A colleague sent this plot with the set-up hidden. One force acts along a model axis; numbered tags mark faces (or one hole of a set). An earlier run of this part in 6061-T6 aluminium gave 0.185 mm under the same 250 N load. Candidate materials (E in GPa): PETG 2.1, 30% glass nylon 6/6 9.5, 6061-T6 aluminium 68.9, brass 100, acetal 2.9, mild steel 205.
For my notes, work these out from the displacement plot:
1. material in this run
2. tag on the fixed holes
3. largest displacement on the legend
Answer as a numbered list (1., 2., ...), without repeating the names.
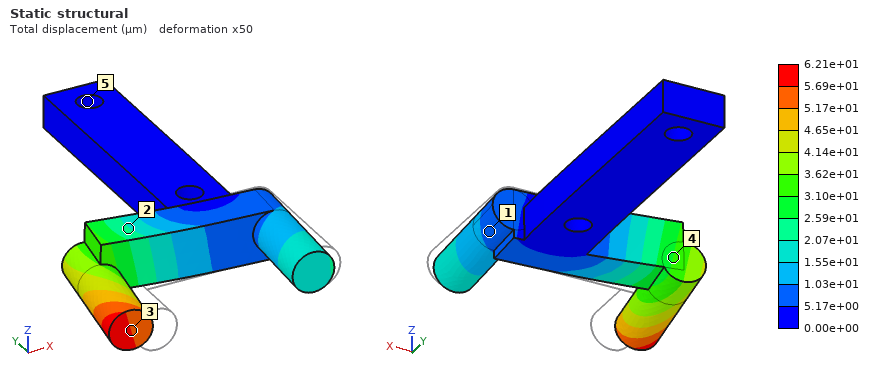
1. mild steel
2. 5
3. 6.21e+01 µm
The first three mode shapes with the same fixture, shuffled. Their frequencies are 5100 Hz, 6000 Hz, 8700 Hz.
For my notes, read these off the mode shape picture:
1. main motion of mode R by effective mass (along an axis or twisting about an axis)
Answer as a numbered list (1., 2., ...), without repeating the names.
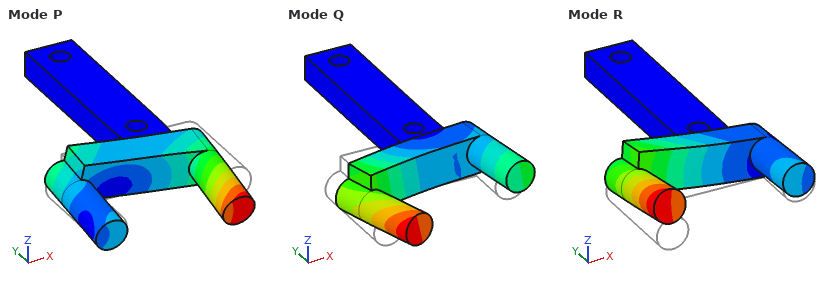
1. along Z
